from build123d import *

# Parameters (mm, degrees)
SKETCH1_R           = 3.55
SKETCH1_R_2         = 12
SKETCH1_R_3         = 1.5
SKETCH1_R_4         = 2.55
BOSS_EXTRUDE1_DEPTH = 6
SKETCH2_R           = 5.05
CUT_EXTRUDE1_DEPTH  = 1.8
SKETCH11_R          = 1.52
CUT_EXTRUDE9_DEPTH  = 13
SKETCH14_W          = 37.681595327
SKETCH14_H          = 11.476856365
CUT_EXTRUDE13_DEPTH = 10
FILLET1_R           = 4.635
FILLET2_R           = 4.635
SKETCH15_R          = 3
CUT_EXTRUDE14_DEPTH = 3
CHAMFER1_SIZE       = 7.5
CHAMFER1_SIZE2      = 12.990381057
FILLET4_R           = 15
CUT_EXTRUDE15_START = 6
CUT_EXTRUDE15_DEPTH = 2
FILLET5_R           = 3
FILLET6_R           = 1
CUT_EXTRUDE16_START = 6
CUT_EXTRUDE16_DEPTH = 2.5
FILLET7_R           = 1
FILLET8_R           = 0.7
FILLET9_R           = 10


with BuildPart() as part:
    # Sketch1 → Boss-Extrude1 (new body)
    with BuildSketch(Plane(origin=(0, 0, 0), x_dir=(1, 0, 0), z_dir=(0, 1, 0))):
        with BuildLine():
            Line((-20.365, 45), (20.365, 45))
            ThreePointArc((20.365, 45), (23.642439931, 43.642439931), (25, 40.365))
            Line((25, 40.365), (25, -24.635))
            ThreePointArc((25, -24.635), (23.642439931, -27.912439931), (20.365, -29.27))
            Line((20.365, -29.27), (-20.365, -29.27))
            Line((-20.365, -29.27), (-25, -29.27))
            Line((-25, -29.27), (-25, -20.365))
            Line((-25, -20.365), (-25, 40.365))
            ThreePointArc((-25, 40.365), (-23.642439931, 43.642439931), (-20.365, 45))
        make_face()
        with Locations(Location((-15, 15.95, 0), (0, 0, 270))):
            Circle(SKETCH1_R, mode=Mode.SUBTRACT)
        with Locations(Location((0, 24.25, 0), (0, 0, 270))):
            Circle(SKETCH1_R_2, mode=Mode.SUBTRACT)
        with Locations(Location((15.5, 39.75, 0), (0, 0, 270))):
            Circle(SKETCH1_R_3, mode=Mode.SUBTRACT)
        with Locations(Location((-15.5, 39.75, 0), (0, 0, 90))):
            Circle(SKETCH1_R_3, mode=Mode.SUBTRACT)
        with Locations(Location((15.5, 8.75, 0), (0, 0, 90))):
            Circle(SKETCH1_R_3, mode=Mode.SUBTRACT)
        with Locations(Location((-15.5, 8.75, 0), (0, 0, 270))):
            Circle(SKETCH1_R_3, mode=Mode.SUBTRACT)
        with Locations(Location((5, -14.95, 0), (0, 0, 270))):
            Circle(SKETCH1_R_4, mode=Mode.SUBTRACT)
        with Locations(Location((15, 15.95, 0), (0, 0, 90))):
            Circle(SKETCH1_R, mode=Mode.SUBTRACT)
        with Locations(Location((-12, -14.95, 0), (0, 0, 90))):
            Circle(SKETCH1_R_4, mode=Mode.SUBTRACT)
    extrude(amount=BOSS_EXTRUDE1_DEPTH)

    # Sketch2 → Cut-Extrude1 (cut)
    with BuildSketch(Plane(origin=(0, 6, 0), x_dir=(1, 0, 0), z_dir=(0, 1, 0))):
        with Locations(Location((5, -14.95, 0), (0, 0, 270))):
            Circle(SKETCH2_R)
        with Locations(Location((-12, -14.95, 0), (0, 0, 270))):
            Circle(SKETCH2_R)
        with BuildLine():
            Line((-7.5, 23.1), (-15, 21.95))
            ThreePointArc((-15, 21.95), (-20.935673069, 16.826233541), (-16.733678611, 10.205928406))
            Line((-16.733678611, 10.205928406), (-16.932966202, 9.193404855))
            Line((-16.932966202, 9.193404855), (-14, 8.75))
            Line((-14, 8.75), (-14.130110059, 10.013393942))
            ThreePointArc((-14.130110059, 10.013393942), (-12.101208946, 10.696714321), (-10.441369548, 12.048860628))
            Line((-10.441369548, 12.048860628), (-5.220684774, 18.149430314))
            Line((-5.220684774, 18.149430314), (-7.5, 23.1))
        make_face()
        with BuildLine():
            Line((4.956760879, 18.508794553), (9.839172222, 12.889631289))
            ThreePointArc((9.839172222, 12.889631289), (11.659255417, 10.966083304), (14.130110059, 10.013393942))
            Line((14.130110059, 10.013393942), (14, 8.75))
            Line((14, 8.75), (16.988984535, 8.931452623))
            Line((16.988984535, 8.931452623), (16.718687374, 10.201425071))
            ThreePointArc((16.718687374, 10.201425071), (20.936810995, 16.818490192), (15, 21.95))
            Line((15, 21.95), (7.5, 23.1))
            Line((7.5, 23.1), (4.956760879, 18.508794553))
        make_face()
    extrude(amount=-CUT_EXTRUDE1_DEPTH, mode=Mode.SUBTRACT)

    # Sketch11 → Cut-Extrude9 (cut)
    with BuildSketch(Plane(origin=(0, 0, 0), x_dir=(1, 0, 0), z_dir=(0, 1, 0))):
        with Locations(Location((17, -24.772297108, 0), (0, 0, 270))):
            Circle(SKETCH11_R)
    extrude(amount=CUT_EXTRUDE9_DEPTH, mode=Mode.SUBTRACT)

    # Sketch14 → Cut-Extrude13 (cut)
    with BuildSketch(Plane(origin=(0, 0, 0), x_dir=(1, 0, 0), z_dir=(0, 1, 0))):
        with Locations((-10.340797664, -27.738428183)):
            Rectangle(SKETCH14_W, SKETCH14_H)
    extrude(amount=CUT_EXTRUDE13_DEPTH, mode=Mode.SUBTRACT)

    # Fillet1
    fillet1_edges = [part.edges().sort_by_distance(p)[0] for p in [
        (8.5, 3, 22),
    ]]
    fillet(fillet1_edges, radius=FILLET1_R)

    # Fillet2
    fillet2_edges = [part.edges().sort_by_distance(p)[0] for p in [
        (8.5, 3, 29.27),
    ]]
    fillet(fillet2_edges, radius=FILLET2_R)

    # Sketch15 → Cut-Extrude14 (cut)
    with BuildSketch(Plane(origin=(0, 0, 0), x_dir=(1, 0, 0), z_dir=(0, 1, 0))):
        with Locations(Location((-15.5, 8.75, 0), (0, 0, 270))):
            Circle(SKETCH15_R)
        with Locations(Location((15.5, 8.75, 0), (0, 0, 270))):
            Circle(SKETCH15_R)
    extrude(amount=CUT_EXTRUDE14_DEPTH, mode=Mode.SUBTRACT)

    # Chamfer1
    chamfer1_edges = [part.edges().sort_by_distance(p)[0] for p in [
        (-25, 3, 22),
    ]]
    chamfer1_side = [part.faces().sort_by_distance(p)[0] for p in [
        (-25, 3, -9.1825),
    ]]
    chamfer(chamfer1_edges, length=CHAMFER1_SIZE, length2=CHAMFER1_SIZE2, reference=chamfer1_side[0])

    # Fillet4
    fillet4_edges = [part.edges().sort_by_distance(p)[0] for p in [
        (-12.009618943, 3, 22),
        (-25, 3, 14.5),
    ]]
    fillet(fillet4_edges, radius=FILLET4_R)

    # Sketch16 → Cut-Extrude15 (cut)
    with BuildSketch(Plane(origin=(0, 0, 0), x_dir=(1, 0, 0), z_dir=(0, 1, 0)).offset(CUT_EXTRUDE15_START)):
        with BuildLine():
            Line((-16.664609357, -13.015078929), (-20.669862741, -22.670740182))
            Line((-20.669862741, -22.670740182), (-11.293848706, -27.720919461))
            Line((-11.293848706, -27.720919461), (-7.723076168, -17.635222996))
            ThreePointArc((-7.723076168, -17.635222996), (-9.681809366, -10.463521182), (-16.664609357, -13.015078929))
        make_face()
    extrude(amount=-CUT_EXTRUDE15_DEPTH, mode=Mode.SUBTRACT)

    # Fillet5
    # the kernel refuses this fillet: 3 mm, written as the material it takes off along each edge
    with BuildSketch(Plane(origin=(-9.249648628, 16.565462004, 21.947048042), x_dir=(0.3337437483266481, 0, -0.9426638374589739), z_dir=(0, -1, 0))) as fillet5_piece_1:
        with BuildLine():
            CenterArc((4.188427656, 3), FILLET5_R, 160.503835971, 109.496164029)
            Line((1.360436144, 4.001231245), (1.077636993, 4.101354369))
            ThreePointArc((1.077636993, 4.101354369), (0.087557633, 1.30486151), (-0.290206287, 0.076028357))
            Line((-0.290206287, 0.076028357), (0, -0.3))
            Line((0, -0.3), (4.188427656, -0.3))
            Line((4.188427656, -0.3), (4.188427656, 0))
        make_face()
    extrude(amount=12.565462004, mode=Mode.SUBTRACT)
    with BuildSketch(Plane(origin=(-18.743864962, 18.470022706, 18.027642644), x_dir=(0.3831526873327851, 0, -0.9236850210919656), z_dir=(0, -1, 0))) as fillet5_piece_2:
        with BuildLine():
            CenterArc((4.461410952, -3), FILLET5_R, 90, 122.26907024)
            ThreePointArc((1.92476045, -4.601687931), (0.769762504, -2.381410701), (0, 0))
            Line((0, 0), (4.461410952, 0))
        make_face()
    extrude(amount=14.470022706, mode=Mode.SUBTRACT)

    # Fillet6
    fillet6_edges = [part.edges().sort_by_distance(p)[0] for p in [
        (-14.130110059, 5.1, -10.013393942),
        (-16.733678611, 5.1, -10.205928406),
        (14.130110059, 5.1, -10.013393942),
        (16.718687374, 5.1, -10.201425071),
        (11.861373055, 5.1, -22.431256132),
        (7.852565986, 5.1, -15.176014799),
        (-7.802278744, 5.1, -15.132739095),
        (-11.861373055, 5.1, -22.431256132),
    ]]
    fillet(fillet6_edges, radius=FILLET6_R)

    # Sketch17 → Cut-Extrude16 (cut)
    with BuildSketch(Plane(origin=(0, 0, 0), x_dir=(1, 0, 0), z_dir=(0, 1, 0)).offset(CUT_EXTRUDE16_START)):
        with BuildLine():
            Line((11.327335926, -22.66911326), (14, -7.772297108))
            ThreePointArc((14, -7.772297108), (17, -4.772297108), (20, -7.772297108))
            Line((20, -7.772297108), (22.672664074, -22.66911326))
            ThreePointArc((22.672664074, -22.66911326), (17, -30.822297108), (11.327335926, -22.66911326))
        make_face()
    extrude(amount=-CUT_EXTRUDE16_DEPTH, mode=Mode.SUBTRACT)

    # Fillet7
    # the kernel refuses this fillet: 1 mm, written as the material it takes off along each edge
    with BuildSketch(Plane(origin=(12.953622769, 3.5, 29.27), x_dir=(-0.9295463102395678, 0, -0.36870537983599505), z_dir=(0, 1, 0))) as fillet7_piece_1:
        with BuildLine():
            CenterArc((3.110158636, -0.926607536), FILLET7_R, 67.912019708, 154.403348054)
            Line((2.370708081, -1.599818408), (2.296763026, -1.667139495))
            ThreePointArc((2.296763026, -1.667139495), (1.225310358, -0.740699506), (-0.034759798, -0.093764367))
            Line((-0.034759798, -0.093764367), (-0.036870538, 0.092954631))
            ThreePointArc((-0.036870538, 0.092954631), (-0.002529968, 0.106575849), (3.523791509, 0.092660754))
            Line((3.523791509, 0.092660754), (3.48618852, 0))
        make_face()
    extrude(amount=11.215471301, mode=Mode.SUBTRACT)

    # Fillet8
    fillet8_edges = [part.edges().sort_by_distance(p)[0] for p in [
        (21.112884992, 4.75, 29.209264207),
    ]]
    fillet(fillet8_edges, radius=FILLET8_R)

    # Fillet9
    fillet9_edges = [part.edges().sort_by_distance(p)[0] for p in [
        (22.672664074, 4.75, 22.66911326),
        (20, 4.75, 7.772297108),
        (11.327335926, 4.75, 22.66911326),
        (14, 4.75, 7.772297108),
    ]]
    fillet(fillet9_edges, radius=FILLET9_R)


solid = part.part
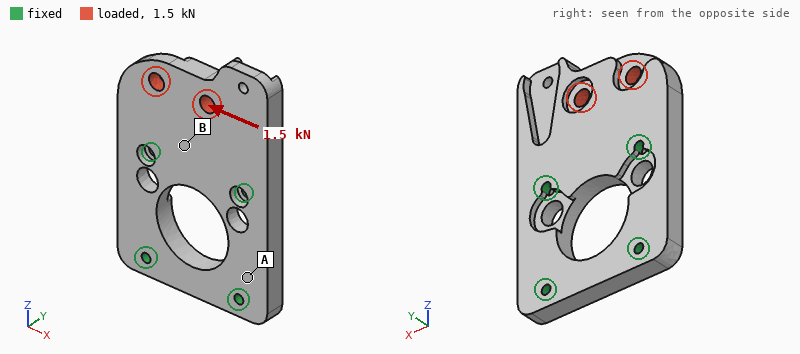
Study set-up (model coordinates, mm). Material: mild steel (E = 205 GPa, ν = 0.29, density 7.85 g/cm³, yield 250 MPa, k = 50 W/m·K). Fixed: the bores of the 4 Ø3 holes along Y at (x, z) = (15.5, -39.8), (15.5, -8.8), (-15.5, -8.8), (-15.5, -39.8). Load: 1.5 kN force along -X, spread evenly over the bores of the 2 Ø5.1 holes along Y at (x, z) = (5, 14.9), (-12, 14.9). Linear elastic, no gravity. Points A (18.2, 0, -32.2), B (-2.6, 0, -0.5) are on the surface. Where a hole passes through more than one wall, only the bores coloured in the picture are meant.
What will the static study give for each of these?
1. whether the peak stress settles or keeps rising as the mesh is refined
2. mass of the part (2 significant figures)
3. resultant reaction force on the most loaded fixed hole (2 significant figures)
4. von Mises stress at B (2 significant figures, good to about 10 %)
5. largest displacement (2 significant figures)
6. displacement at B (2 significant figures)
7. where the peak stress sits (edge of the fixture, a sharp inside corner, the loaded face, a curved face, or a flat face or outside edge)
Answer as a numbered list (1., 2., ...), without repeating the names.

1. keeps rising
2. 120 g
3. 1.1 kN
4. 12 MPa
5. 5.2 µm
6. 1.5 µm
7. edge of the fixture
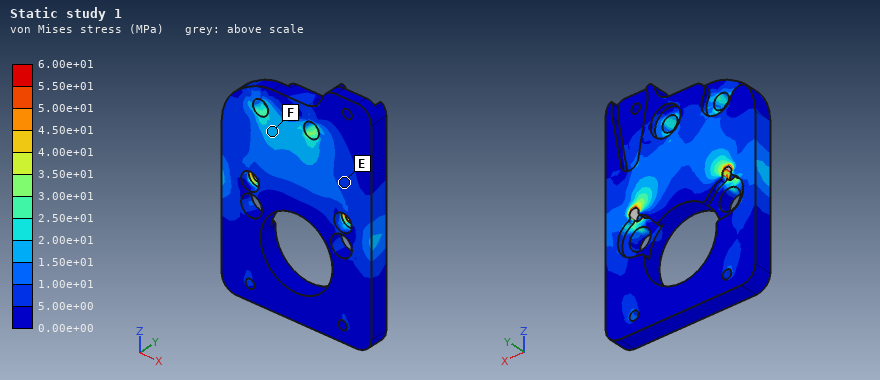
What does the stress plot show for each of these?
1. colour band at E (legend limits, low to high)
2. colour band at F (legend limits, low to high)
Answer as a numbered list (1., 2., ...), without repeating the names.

1. 5.00e+00 to 1.00e+01 MPa
2. 1.50e+01 to 2.00e+01 MPa
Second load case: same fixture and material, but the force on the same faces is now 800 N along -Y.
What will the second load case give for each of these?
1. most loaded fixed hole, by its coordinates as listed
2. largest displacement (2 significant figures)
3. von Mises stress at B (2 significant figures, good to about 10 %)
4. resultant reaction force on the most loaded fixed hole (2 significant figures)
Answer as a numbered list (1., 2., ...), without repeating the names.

1. (-15.5, -8.8)
2. 85 µm
3. 41 MPa
4. 950 N
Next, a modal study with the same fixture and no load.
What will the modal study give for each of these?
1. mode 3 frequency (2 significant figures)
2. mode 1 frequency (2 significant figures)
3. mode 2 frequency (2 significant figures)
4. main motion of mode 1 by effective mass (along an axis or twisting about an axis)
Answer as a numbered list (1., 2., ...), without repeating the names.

1. 14 kHz
2. 3200 Hz
3. 7200 Hz
4. along Y
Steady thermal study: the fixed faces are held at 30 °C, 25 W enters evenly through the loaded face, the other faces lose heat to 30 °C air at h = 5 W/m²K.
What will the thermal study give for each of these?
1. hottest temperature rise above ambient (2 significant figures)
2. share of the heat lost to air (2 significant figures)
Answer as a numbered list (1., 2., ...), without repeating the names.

1. 75 K
2. 3.7 %
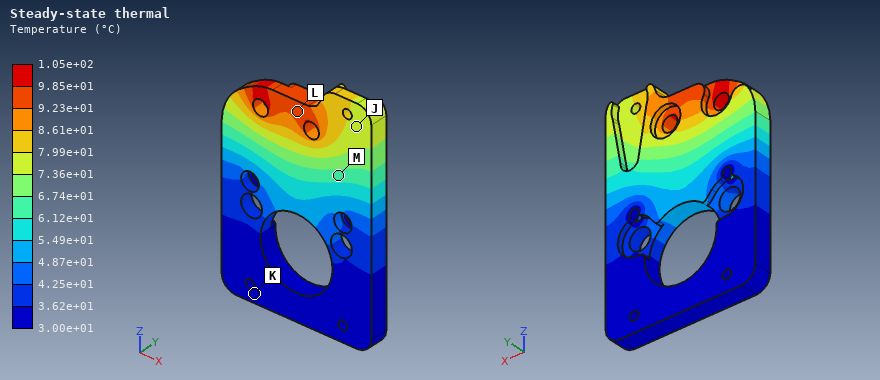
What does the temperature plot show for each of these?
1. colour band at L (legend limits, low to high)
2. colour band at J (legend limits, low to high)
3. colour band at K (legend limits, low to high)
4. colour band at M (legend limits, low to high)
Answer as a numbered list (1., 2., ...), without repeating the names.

1. 9.23e+01 to 9.85e+01 °C
2. 7.36e+01 to 7.99e+01 °C
3. 3.00e+01 to 3.62e+01 °C
4. 6.12e+01 to 6.74e+01 °C
